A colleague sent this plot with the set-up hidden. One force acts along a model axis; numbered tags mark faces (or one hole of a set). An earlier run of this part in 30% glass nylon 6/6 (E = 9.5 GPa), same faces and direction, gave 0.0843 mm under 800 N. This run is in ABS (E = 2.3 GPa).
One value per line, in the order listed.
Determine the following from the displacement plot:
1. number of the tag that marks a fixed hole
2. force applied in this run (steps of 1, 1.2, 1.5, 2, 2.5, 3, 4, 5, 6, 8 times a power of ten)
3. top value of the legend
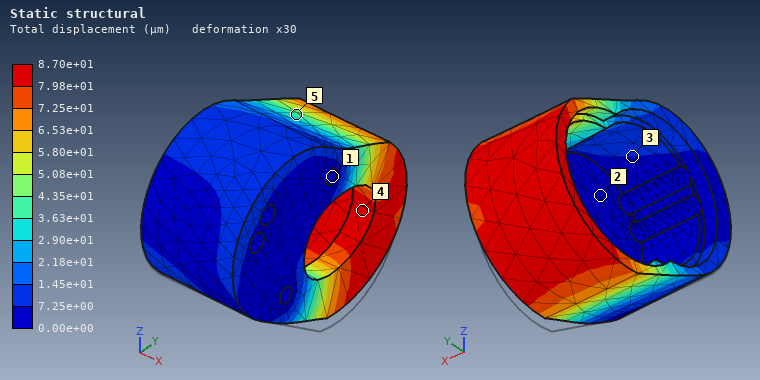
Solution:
1
200 N
8.70e+01 µm
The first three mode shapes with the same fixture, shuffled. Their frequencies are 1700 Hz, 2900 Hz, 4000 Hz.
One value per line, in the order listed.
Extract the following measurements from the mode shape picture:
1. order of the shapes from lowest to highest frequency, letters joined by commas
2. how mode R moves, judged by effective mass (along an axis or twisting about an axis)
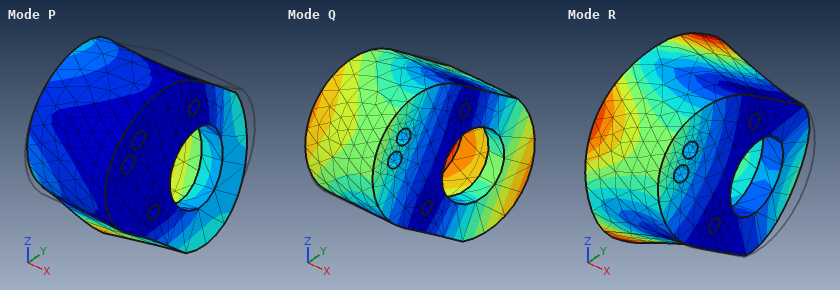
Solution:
Q, P, R
along X
